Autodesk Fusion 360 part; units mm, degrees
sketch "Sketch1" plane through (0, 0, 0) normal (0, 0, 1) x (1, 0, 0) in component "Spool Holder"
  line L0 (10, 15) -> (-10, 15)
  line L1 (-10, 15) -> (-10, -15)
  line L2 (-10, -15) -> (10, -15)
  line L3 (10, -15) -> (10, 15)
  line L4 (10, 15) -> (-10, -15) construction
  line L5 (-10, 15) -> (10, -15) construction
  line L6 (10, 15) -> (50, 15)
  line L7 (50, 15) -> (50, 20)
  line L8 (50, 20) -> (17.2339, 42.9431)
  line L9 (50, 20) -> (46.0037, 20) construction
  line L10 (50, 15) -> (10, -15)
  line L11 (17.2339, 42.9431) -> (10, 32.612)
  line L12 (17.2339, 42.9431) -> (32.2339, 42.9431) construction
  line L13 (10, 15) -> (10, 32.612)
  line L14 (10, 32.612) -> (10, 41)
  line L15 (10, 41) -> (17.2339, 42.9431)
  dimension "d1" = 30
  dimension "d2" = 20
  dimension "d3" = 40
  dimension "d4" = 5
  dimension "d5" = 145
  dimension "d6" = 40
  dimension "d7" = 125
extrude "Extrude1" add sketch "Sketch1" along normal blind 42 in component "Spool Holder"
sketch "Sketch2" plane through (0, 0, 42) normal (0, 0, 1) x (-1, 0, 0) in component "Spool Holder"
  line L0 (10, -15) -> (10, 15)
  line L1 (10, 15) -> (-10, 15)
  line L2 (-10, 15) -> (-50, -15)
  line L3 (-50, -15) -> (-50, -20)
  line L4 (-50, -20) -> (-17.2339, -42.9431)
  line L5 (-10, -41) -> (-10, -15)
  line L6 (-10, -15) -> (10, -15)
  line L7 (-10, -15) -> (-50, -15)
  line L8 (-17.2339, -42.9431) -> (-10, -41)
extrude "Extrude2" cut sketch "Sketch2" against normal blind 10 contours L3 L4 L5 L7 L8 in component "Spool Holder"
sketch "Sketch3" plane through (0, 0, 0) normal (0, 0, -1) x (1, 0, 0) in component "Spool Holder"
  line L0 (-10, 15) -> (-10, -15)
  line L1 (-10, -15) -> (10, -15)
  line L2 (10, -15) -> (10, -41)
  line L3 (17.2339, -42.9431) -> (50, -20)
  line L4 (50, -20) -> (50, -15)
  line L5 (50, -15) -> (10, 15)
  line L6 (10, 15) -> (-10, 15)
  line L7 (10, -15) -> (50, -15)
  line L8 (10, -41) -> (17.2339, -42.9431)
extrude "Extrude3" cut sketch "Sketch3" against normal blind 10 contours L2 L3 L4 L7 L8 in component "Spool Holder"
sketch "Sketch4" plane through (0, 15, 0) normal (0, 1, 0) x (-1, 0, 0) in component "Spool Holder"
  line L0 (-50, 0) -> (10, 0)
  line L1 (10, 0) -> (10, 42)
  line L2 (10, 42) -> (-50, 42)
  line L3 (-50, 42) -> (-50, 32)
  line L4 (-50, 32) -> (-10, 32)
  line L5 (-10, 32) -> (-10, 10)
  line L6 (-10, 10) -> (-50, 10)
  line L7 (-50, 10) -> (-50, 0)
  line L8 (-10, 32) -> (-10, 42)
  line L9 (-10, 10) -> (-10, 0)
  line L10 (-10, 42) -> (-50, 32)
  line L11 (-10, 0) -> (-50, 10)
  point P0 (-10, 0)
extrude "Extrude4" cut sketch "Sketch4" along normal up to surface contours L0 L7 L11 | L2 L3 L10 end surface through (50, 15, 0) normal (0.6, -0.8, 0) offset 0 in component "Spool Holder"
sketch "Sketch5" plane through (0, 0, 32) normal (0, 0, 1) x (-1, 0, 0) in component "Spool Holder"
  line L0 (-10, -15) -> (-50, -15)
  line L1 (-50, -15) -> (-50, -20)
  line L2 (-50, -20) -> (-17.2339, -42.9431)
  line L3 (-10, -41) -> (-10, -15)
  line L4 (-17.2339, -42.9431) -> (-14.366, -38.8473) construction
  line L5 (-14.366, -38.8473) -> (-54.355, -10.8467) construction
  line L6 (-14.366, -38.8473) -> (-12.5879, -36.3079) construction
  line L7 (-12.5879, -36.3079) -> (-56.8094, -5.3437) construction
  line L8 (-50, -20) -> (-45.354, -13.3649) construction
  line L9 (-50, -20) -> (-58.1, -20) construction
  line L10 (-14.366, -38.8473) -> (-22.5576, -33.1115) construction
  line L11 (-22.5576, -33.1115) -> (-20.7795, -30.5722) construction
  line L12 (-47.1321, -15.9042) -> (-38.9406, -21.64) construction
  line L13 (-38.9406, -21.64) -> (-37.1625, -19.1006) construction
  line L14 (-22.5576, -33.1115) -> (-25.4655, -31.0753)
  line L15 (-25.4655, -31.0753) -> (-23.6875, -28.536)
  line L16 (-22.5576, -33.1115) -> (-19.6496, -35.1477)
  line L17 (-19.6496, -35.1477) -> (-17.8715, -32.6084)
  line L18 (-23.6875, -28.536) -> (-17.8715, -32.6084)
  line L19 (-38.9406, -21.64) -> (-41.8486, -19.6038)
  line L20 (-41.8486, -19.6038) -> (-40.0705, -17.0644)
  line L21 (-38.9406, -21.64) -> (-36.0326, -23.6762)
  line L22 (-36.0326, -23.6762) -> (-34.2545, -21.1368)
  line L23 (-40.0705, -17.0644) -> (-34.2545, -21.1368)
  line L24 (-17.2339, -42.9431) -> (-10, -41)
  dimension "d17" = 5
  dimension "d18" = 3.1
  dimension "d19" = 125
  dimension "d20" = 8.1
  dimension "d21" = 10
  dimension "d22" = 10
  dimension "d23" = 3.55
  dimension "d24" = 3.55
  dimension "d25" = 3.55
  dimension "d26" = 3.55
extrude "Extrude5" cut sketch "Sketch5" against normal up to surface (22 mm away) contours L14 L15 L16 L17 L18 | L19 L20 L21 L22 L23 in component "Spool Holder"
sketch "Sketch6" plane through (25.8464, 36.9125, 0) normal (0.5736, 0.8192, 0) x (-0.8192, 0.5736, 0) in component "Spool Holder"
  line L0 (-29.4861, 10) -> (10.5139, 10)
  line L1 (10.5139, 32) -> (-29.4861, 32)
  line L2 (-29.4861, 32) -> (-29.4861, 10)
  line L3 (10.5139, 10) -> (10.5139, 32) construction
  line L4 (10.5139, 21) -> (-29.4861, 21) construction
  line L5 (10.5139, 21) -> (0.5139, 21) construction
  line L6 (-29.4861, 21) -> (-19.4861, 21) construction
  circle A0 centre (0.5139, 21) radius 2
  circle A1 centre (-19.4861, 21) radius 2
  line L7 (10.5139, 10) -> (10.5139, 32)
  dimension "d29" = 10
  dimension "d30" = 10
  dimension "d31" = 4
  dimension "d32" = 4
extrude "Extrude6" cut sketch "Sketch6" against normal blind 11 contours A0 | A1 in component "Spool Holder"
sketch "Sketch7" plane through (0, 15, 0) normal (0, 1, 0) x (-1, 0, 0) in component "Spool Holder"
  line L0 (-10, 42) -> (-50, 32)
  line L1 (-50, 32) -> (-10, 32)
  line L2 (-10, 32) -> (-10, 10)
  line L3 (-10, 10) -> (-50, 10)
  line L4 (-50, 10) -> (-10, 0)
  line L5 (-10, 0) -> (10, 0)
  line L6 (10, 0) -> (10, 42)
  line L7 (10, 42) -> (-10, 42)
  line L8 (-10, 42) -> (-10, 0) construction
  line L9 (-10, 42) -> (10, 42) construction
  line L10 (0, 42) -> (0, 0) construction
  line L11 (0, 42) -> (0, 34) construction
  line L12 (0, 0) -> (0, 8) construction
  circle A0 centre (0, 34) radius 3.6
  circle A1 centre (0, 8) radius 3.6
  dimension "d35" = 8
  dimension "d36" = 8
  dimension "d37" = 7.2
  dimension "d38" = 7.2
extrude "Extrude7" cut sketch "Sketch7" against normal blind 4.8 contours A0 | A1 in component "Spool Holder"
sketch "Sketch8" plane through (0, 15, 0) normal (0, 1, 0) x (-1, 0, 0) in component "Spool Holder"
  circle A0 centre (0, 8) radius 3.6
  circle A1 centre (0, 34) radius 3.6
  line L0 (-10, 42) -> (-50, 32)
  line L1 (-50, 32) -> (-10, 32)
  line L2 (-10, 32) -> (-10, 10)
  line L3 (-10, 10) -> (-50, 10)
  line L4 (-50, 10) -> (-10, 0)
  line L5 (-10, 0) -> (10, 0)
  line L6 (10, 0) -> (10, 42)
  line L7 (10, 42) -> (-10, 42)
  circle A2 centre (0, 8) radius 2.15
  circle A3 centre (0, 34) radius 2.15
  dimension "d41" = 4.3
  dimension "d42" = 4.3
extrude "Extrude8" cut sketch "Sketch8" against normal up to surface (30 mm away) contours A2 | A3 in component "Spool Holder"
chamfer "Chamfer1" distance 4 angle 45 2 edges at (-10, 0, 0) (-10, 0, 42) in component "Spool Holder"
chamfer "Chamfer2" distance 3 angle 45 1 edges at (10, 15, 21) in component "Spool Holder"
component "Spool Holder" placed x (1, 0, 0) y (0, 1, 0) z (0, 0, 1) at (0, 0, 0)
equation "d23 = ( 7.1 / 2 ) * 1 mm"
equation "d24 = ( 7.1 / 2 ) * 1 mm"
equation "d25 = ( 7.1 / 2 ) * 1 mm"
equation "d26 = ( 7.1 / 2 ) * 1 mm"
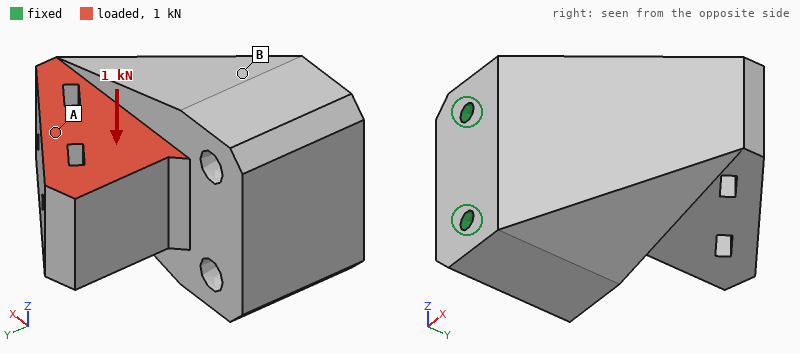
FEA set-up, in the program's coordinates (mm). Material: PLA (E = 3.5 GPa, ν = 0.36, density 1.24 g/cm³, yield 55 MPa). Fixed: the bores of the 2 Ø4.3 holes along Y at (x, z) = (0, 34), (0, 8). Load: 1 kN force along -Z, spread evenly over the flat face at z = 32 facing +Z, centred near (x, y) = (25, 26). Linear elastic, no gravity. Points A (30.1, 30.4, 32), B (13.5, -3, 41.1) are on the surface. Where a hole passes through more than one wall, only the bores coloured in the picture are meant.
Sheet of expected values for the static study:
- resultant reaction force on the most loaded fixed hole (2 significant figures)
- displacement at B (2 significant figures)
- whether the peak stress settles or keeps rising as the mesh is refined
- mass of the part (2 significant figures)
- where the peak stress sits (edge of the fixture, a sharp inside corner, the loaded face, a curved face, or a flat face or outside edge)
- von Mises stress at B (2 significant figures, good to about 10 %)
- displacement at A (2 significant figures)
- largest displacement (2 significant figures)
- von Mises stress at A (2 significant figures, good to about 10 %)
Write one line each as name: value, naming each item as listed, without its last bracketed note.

resultant reaction force on the most loaded fixed hole: 1.2 kN
displacement at B: 0.025 mm
whether the peak stress settles or keeps rising as the mesh is refined: keeps rising
mass of the part: 74 g
where the peak stress sits: edge of the fixture
von Mises stress at B: 3.4 MPa
displacement at A: 0.12 mm
largest displacement: 0.16 mm
von Mises stress at A: 1.7 MPa
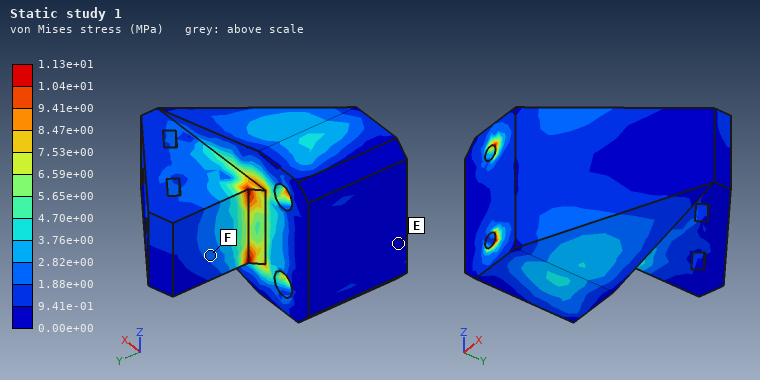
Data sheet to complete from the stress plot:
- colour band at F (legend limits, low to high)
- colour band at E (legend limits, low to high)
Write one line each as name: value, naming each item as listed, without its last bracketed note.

colour band at F: 1.88e+00 to 2.82e+00 MPa
colour band at E: 0.00e+00 to 9.41e-01 MPa
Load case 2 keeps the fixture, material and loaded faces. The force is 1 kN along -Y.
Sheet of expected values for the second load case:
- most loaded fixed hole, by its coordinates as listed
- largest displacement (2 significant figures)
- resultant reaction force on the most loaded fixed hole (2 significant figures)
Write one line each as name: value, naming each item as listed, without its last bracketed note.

most loaded fixed hole, by its coordinates as listed: (0, 34)
largest displacement: 0.18 mm
resultant reaction force on the most loaded fixed hole: 780 N
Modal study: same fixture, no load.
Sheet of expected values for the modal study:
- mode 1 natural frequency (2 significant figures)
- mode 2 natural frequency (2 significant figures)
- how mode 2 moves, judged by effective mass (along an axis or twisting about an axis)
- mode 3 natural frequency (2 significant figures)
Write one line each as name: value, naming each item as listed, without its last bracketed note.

mode 1 natural frequency: 2300 Hz
mode 2 natural frequency: 3200 Hz
how mode 2 moves, judged by effective mass: along Z
mode 3 natural frequency: 4800 Hz
